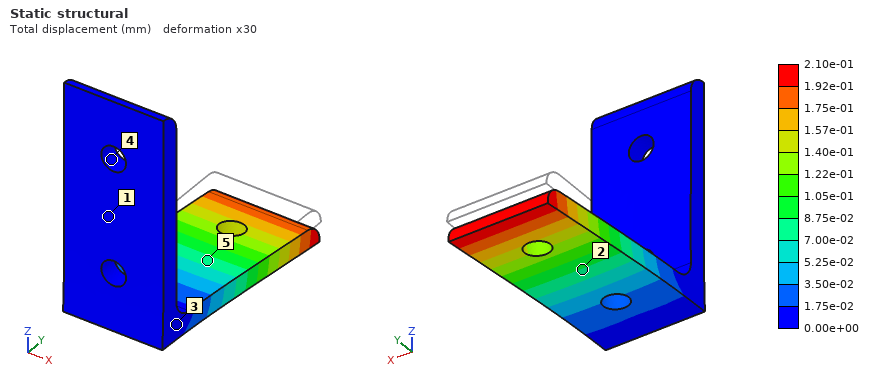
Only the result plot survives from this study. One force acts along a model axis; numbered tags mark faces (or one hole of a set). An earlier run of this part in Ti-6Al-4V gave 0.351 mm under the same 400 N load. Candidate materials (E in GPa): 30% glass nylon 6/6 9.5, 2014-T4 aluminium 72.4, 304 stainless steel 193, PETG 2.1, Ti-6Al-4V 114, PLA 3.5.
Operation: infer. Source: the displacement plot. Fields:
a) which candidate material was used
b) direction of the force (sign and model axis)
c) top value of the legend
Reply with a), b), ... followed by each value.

a) 304 stainless steel
b) -Z
c) 2.10e-01 mm
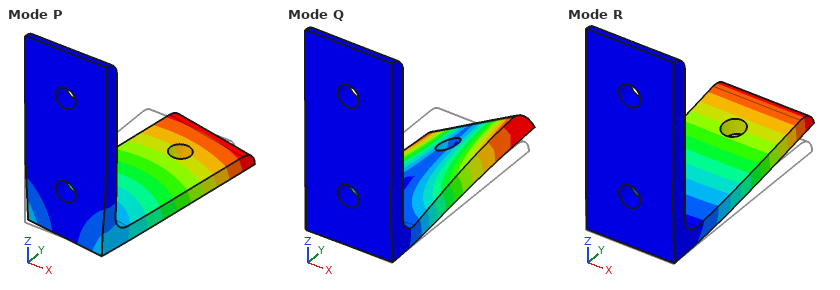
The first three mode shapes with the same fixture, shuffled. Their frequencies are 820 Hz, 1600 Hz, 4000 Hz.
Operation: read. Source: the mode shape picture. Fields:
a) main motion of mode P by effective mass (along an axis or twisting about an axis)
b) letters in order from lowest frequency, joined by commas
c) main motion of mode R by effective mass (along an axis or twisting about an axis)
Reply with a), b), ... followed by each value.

a) along X
b) R, P, Q
c) along Z
